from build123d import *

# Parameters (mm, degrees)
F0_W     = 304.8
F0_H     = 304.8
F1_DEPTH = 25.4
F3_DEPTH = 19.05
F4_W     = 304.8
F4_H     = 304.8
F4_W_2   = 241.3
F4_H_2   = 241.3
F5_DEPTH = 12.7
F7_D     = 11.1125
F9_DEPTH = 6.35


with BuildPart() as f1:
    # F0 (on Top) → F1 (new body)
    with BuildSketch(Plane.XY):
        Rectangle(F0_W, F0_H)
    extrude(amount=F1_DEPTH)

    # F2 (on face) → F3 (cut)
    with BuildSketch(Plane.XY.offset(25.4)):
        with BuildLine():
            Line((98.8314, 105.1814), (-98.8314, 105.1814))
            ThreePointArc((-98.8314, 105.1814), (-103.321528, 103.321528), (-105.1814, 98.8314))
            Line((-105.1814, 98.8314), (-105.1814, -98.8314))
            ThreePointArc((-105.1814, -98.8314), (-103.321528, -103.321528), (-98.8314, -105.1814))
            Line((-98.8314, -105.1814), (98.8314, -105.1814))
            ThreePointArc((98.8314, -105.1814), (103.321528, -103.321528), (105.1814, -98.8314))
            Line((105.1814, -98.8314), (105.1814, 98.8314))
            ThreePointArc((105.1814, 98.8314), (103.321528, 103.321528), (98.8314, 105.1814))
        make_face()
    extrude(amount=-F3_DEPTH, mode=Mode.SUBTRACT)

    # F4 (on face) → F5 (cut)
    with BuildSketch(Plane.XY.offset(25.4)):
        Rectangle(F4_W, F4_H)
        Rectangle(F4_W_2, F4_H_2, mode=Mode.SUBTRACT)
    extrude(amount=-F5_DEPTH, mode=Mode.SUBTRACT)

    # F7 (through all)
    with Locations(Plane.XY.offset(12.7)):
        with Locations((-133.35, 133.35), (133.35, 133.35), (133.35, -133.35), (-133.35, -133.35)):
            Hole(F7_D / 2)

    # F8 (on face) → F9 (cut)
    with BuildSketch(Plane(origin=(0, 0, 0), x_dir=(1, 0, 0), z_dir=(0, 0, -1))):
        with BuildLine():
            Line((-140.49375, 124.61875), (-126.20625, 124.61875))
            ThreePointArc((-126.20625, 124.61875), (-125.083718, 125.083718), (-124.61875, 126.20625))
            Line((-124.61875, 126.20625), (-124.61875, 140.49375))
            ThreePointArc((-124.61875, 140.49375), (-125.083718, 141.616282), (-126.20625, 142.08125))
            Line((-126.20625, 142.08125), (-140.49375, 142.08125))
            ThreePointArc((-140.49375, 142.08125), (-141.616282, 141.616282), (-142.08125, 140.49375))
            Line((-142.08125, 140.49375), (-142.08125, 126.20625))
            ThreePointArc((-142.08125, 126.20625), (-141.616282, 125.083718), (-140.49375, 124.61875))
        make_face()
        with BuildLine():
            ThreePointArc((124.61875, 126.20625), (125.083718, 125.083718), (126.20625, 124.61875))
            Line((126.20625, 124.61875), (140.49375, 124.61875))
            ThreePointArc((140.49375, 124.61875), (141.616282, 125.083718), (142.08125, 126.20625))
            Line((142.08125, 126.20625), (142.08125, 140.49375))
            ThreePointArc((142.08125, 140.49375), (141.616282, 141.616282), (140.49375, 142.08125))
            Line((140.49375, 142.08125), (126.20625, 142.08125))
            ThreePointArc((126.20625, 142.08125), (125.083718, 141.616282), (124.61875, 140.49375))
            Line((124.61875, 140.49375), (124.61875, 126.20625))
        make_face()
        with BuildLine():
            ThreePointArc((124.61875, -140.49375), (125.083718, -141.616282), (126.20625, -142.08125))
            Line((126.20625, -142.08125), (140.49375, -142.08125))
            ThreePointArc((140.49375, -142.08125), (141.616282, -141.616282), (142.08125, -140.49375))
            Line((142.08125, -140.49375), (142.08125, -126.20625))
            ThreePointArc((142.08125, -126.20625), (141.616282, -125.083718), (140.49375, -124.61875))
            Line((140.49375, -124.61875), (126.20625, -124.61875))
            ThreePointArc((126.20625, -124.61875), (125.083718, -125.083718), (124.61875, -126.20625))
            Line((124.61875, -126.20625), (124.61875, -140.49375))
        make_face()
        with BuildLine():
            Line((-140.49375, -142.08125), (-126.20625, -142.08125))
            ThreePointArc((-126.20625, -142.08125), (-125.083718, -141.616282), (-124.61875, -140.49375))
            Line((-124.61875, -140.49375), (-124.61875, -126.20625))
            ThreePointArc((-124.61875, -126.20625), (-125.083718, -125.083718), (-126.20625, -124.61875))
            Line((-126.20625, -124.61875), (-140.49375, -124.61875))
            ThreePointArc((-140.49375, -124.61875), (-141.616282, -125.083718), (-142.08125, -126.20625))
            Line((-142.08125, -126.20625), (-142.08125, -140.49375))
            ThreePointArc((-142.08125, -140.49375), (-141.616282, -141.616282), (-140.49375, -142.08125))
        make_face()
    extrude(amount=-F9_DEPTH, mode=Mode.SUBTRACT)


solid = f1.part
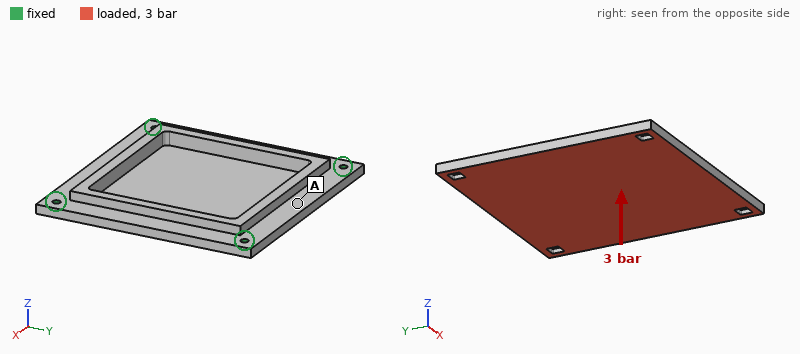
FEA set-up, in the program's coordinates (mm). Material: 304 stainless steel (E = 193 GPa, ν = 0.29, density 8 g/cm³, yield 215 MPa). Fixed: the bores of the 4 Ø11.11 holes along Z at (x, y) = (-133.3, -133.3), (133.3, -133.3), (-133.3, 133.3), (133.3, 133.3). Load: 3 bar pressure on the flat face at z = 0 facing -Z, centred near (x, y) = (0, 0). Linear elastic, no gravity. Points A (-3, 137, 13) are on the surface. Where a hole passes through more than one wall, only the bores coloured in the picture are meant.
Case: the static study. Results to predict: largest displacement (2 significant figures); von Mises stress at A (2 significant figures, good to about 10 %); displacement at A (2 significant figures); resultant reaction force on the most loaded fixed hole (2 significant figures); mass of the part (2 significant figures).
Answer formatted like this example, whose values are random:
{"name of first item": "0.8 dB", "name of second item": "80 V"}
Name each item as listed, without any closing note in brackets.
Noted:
{"largest displacement": "0.56 mm", "von Mises stress at A": "30 MPa", "displacement at A": "0.17 mm", "resultant reaction force on the most loaded fixed hole": "10 kN", "mass of the part": "8.5 kg"}
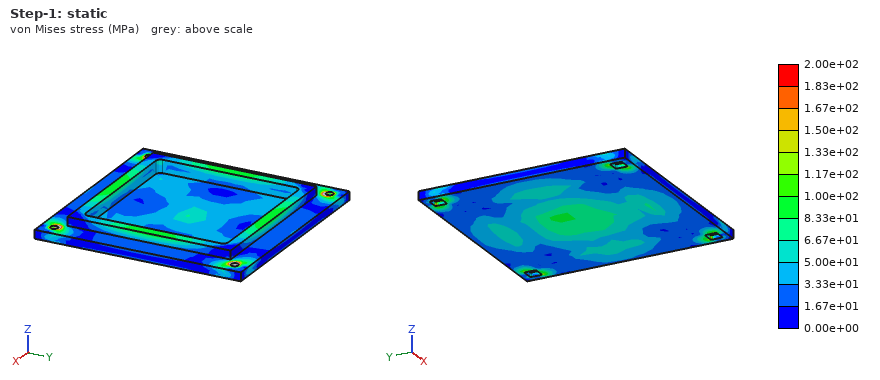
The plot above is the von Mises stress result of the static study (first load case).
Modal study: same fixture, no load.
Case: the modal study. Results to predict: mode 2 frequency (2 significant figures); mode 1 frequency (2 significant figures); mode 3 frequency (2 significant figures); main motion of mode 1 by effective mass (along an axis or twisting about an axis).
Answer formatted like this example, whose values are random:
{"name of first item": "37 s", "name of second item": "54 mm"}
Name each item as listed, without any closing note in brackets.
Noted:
{"mode 2 frequency": "950 Hz", "mode 1 frequency": "600 Hz", "mode 3 frequency": "960 Hz", "main motion of mode 1 by effective mass": "along Z"}
